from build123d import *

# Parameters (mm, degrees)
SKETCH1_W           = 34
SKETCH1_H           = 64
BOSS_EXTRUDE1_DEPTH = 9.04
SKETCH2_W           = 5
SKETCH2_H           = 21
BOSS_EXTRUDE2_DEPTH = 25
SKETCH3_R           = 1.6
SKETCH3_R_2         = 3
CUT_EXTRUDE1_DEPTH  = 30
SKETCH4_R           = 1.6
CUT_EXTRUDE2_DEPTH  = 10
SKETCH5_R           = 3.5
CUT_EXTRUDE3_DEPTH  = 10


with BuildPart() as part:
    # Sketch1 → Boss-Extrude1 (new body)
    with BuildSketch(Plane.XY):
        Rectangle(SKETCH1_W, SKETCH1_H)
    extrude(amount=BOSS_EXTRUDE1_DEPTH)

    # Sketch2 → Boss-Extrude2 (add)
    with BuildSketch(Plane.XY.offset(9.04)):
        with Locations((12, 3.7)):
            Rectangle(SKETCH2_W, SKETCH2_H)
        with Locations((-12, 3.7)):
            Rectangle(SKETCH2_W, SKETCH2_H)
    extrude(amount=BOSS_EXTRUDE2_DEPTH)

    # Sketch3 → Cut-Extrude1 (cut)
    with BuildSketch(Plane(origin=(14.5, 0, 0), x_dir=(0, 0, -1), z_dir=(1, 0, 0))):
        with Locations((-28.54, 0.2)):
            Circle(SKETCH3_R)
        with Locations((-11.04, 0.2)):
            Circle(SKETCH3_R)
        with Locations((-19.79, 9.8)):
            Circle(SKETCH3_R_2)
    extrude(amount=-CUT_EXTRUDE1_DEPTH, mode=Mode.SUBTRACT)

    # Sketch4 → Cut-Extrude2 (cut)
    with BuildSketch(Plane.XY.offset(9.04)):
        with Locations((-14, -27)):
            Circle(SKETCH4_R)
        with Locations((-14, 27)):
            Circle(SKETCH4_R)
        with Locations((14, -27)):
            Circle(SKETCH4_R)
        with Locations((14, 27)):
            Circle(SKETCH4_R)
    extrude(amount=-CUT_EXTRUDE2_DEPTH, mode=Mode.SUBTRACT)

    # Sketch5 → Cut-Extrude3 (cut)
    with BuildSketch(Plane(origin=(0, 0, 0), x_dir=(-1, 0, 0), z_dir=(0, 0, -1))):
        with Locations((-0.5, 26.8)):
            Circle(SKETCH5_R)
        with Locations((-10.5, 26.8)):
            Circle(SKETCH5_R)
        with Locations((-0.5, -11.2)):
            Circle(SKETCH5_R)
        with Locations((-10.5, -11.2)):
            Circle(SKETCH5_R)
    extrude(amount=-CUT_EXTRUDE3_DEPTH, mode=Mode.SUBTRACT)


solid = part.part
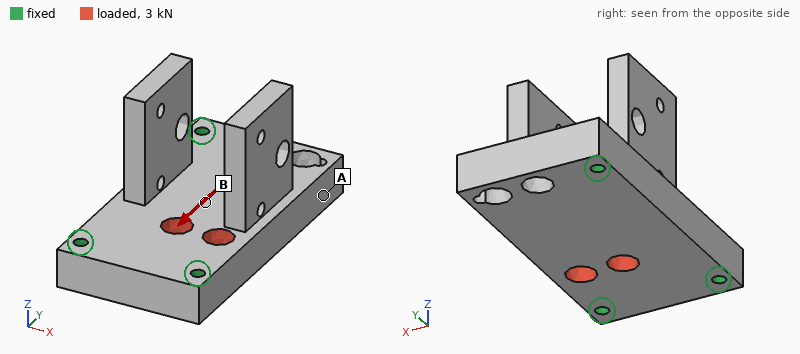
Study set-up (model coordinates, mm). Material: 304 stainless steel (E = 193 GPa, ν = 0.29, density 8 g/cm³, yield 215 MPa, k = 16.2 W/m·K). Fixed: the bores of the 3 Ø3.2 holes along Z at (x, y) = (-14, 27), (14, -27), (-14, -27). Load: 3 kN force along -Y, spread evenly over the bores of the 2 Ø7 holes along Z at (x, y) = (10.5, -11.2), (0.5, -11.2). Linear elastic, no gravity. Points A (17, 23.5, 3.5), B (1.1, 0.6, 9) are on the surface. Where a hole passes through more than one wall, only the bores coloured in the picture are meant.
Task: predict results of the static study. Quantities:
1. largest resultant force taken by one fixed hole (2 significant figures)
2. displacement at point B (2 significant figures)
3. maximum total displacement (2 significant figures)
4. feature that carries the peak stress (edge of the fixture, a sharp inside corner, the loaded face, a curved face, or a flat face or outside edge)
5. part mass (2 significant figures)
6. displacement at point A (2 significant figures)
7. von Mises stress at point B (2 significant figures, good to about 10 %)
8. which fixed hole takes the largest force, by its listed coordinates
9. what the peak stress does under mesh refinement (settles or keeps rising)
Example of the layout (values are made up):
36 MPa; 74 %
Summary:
1.4 kN; 1.1 µm; 1.6 µm; edge of the fixture; 180 g; 1.4 µm; 5.8 MPa; (14, -27); keeps rising
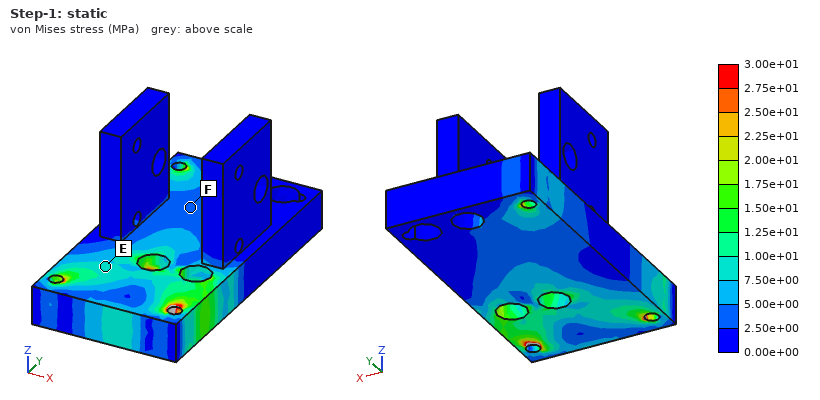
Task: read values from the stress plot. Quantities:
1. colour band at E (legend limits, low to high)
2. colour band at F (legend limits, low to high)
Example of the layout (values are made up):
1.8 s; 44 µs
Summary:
7.50e+00 to 1.00e+01 MPa; 2.50e+00 to 5.00e+00 MPa
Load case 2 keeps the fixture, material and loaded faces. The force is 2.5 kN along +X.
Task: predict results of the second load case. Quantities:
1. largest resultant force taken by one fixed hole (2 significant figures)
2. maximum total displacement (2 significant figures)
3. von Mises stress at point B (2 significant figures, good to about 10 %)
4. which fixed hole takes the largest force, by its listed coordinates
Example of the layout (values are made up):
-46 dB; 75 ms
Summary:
1.3 kN; 2.6 µm; 3.5 MPa; (-14, -27)
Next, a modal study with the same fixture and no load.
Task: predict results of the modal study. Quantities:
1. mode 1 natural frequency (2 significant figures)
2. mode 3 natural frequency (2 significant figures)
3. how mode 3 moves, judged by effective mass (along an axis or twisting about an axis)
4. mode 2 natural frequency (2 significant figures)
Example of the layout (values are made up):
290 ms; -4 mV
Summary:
4100 Hz; 6400 Hz; along Z; 4900 Hz
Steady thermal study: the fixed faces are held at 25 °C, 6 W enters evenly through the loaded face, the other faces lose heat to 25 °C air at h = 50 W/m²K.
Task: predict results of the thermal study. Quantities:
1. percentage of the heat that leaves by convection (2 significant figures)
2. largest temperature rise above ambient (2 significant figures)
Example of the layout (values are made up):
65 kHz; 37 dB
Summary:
38 %; 17 K
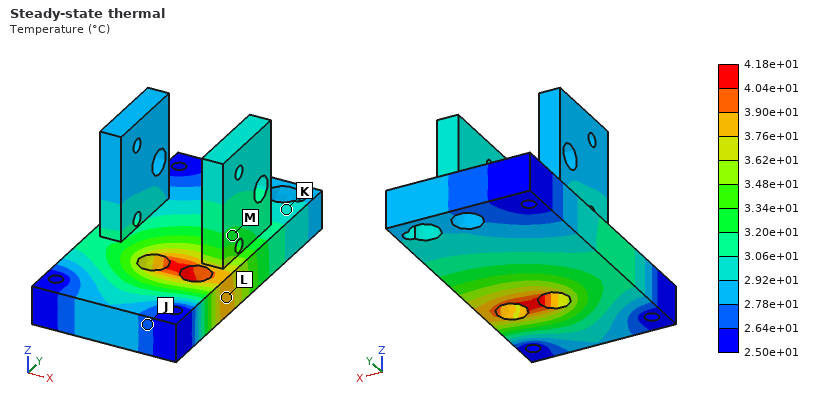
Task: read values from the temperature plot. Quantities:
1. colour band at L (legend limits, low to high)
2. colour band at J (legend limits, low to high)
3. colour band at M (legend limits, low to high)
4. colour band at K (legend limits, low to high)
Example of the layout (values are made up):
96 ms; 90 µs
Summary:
3.76e+01 to 3.90e+01 °C; 2.64e+01 to 2.78e+01 °C; 3.20e+01 to 3.34e+01 °C; 2.92e+01 to 3.06e+01 °C
